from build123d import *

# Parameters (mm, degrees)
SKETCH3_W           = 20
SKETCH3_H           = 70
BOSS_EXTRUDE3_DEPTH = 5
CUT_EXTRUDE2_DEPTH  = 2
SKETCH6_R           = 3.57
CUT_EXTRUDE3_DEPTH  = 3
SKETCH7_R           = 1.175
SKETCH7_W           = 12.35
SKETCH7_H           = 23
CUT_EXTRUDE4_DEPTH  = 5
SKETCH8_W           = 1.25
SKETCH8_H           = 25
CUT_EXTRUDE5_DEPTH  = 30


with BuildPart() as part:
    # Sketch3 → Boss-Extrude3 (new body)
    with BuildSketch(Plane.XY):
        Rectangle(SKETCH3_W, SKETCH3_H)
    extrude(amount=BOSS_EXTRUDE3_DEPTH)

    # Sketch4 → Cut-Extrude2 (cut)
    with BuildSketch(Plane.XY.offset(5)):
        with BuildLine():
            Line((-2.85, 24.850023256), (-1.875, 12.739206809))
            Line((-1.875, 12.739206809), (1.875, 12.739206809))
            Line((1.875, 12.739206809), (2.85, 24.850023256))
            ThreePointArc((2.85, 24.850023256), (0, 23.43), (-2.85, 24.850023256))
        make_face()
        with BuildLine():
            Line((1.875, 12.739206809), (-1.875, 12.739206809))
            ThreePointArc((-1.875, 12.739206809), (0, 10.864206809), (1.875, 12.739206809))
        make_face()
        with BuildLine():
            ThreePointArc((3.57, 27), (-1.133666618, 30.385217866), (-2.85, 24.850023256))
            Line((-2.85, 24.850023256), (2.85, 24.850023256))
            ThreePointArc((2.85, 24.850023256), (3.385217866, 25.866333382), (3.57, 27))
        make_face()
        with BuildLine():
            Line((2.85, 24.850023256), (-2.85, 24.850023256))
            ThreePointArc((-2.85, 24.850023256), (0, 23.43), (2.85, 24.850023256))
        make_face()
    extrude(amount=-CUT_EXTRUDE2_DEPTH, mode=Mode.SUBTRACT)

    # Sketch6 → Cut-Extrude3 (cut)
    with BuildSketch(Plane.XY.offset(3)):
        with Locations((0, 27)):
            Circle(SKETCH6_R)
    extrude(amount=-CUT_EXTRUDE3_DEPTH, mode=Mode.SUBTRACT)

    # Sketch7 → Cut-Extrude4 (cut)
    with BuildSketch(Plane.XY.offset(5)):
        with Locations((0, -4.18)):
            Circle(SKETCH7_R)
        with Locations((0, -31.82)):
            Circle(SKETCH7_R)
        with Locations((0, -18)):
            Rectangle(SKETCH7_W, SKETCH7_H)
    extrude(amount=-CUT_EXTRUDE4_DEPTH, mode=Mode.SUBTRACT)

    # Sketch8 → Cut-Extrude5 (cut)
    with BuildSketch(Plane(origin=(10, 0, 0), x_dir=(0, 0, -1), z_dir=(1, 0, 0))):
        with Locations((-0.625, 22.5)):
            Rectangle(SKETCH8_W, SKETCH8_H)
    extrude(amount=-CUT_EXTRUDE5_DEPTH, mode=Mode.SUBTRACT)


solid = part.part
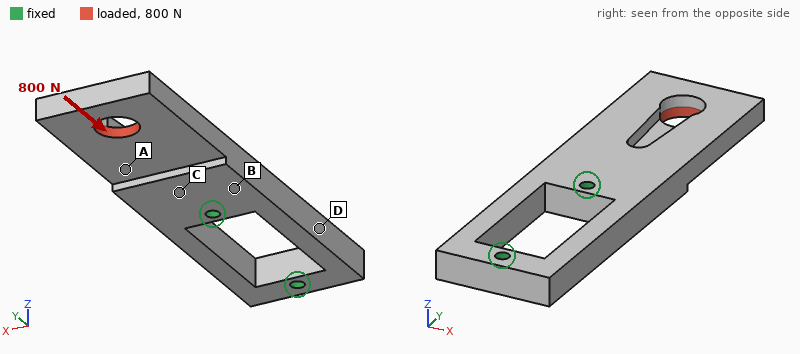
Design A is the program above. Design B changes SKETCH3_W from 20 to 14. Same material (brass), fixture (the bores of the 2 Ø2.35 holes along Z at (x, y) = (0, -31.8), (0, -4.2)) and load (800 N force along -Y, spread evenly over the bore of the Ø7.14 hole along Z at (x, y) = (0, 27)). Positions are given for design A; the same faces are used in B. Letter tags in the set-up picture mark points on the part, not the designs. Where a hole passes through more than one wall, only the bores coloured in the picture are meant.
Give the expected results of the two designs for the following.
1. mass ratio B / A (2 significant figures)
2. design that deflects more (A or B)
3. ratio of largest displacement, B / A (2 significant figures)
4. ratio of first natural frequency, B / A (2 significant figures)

0.59
B
1.5
1.1
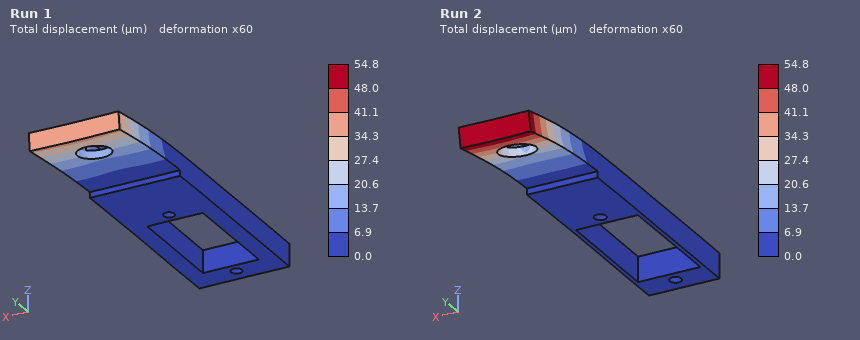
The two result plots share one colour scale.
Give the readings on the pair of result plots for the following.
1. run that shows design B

Run 2
